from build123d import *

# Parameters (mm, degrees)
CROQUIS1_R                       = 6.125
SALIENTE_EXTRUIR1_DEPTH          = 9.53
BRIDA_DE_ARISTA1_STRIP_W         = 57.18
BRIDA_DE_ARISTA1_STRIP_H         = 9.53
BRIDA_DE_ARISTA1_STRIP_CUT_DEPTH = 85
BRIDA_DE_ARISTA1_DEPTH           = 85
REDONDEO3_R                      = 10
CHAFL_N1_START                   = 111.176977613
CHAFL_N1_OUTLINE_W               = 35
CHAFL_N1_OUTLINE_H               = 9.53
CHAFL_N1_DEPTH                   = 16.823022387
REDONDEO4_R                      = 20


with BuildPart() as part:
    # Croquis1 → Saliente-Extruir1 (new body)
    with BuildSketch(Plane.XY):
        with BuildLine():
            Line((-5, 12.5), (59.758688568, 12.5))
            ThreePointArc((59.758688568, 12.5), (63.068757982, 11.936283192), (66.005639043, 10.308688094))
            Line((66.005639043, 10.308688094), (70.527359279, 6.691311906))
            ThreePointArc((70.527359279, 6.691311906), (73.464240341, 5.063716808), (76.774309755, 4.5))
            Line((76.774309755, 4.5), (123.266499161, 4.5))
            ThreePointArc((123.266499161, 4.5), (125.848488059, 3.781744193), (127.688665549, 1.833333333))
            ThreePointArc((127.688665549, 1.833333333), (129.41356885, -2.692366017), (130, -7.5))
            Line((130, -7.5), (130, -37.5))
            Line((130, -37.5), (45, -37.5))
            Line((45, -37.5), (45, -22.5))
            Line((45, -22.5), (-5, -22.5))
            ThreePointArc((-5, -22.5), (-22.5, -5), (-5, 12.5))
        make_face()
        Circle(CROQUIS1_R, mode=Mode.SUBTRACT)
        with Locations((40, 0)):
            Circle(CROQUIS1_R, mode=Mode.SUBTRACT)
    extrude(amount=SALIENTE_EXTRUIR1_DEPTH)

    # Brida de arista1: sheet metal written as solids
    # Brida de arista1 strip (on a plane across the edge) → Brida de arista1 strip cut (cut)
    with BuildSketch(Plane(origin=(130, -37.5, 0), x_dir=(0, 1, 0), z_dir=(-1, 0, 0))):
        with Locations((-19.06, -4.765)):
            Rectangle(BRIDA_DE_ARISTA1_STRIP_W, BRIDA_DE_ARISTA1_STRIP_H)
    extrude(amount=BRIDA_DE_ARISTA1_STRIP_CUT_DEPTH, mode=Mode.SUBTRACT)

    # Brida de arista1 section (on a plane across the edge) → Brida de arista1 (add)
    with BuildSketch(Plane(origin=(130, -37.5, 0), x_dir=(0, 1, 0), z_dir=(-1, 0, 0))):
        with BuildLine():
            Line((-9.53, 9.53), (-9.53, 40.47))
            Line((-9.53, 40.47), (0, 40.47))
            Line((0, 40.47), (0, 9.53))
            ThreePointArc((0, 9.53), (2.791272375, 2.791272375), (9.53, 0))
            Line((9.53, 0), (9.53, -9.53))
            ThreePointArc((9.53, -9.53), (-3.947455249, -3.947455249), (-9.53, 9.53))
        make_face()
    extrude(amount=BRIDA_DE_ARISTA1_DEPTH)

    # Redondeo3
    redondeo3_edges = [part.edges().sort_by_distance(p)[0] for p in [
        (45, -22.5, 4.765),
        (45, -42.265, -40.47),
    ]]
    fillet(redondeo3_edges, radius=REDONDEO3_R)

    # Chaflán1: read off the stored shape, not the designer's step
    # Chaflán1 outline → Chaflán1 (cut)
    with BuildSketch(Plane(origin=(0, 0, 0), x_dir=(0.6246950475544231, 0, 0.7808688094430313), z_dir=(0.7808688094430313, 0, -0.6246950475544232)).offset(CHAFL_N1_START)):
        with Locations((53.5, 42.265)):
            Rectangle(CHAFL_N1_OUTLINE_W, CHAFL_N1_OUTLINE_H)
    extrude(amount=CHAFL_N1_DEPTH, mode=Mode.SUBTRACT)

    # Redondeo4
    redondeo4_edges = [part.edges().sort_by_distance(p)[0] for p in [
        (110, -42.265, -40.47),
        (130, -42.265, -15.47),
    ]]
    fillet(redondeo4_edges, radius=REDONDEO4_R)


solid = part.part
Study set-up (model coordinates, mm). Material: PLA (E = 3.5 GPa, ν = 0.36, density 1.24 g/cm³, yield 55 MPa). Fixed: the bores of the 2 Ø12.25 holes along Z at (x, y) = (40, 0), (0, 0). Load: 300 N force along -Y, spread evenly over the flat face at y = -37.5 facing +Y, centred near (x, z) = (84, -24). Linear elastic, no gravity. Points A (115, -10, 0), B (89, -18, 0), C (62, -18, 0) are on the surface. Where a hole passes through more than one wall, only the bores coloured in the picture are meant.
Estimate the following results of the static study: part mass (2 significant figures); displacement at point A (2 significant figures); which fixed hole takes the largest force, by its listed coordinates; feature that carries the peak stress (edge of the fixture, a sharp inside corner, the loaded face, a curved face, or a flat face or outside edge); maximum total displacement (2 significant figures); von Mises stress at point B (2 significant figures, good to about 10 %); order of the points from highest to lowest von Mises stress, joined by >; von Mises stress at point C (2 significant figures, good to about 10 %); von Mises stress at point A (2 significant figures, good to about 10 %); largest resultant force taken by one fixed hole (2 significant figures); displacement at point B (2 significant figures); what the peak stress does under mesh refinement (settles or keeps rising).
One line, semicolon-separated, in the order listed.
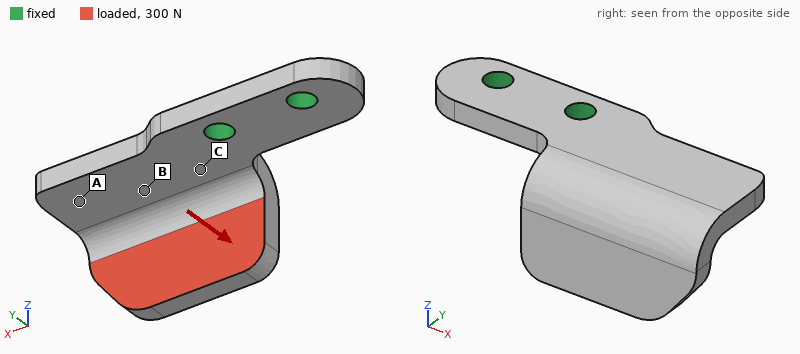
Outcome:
110 g; 0.35 mm; (40, 0); edge of the fixture; 1.9 mm; 6.5 MPa; C > B > A; 11 MPa; 2.9 MPa; 480 N; 0.35 mm; keeps rising
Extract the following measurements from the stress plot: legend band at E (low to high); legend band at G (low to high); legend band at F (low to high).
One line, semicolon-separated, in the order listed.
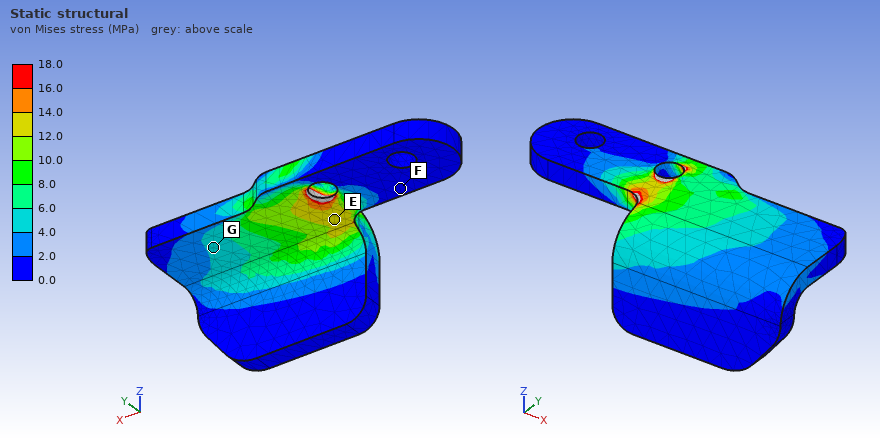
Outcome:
12.0 to 14.0 MPa; 4.0 to 6.0 MPa; 0.0 to 2.0 MPa
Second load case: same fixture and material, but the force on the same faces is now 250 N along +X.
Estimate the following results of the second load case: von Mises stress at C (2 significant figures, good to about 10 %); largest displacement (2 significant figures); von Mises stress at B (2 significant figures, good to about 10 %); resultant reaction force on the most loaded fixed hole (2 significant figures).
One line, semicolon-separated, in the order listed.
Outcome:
8.2 MPa; 1.8 mm; 2.2 MPa; 190 N
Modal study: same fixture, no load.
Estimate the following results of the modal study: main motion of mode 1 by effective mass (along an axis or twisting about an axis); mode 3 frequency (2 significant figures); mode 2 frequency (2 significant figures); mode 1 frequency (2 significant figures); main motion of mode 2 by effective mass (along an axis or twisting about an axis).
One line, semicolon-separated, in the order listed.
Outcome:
along Z; 730 Hz; 430 Hz; 220 Hz; along Y
